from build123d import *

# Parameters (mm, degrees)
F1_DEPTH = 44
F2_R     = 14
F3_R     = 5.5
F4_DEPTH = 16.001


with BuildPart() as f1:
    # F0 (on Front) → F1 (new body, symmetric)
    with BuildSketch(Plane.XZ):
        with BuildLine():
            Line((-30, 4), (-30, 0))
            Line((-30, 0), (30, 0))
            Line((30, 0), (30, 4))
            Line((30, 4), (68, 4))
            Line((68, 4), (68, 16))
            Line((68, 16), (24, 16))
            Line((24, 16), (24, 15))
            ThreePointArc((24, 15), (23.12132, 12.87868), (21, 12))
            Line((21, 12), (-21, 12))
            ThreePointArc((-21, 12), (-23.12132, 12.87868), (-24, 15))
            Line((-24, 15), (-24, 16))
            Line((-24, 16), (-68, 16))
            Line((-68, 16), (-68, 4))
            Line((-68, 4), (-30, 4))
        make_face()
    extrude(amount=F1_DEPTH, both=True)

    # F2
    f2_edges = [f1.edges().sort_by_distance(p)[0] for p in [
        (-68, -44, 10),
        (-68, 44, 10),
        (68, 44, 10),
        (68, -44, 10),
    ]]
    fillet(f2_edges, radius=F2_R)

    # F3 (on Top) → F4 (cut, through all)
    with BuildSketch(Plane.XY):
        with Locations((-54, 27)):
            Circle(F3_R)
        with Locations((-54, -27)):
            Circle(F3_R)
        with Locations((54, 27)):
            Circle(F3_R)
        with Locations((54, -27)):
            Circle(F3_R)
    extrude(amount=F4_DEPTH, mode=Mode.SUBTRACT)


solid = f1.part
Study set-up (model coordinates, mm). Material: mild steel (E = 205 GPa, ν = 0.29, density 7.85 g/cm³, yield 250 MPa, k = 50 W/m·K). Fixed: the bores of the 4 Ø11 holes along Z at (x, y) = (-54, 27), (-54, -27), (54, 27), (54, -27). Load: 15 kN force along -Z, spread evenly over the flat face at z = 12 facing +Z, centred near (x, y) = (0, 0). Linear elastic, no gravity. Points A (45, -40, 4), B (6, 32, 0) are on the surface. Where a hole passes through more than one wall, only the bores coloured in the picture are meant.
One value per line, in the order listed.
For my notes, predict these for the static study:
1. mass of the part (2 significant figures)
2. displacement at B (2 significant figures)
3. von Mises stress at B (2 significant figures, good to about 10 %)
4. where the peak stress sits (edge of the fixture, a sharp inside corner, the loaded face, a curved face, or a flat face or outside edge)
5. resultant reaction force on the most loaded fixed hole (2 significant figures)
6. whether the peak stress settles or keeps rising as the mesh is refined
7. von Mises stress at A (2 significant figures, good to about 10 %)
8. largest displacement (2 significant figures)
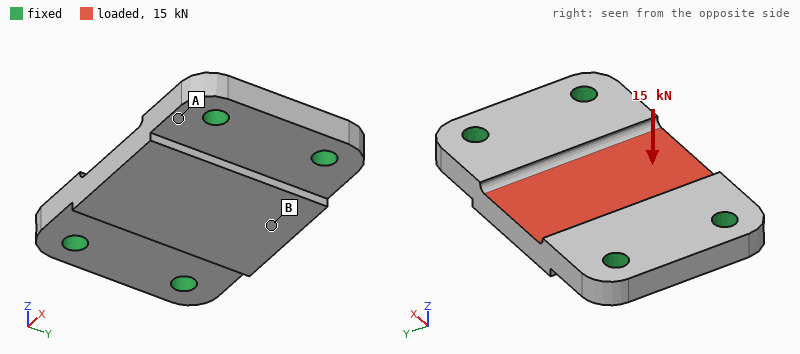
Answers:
1.1 kg
29 µm
59 MPa
edge of the fixture
6.3 kN
keeps rising
32 MPa
32 µm
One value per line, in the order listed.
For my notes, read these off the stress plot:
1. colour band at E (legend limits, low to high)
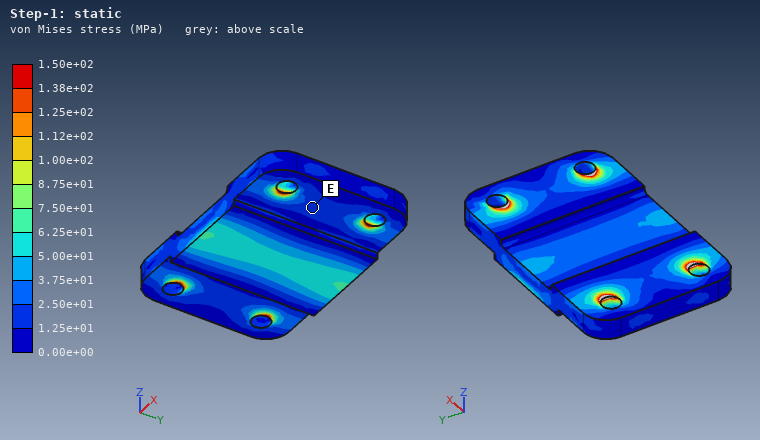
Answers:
1.25e+01 to 2.50e+01 MPa
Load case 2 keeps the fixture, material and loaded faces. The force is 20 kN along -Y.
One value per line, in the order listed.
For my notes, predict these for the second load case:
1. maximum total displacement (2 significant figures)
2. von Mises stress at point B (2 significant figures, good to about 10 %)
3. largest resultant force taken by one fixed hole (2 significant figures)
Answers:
11 µm
16 MPa
5.8 kN
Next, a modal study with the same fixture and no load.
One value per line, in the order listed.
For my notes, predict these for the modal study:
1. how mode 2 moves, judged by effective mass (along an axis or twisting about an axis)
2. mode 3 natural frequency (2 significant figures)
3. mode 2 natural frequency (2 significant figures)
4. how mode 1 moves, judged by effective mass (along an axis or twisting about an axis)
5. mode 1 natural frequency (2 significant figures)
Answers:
twisting about X
12 kHz
6800 Hz
along Z
5400 Hz
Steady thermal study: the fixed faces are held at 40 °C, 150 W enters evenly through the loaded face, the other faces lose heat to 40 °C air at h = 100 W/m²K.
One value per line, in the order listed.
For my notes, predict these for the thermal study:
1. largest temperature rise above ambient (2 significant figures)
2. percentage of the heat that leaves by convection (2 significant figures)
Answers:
53 K
33 %
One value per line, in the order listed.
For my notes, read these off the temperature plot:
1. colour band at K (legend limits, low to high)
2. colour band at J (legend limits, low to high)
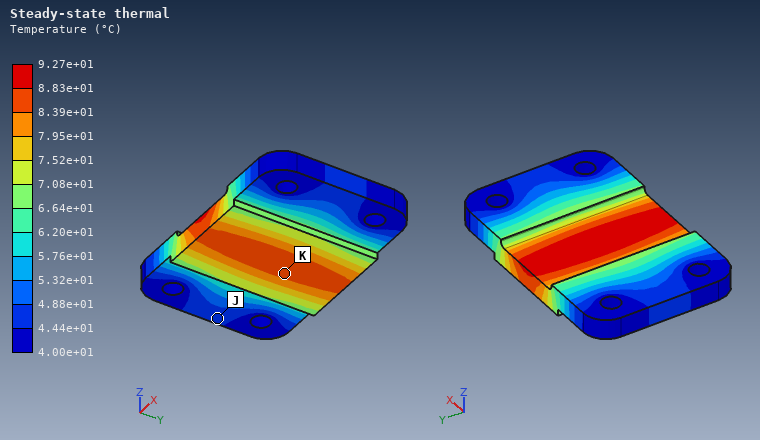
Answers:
8.39e+01 to 8.83e+01 °C
4.44e+01 to 4.88e+01 °C
